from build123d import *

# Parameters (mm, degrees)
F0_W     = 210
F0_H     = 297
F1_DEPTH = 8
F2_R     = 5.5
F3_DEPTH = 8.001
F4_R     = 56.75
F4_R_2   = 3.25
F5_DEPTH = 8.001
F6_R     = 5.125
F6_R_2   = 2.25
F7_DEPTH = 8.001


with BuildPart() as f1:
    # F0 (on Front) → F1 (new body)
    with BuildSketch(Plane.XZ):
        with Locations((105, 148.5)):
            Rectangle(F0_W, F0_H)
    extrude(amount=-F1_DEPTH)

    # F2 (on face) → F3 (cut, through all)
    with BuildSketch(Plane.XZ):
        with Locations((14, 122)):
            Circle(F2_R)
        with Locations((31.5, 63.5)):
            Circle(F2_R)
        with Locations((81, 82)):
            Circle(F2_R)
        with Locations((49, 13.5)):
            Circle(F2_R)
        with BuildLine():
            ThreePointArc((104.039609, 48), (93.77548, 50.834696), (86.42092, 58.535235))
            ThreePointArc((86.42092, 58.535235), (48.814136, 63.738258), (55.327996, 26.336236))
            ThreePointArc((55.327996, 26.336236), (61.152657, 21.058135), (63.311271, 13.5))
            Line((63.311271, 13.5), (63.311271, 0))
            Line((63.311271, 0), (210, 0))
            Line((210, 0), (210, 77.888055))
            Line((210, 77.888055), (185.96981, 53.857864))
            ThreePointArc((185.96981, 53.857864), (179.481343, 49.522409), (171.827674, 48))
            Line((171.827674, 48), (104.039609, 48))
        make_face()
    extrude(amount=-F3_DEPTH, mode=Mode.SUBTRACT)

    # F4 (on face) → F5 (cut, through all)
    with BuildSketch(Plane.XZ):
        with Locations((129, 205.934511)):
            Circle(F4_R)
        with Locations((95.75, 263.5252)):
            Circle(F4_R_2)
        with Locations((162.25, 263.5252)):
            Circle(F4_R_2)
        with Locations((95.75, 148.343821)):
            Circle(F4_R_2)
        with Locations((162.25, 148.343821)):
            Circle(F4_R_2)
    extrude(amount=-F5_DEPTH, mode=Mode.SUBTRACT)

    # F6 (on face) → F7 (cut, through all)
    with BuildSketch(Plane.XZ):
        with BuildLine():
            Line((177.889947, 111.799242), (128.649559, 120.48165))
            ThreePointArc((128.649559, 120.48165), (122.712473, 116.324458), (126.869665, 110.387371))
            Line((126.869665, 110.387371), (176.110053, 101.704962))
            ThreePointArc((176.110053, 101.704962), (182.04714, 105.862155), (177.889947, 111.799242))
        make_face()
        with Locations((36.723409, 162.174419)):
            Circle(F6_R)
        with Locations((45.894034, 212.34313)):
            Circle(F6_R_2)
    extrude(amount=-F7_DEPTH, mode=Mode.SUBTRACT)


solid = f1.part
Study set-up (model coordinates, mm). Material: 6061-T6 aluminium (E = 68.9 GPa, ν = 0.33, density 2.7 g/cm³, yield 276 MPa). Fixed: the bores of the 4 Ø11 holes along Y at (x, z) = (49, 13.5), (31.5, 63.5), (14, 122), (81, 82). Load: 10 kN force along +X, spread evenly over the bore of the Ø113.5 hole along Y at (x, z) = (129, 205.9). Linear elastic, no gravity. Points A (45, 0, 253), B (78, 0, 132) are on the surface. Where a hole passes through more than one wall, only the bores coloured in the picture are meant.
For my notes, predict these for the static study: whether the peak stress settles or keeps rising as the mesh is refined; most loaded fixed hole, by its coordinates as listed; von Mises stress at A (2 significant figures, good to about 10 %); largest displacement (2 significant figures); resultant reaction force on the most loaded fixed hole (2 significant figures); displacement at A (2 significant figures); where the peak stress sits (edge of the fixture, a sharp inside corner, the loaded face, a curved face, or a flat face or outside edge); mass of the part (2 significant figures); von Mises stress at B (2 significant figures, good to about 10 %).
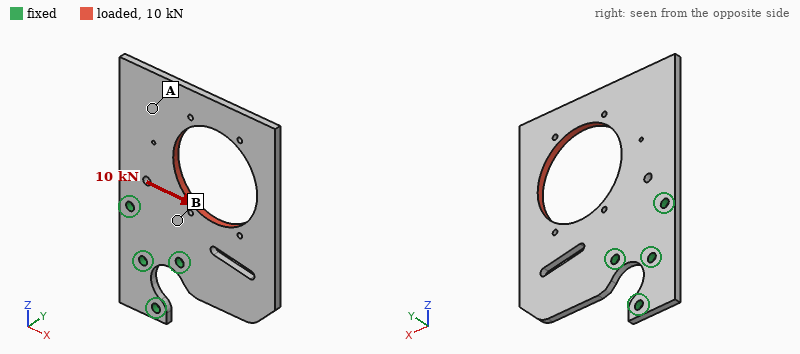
keeps rising
(14, 122)
9.8 MPa
0.32 mm
15 kN
0.21 mm
edge of the fixture
910 g
42 MPa
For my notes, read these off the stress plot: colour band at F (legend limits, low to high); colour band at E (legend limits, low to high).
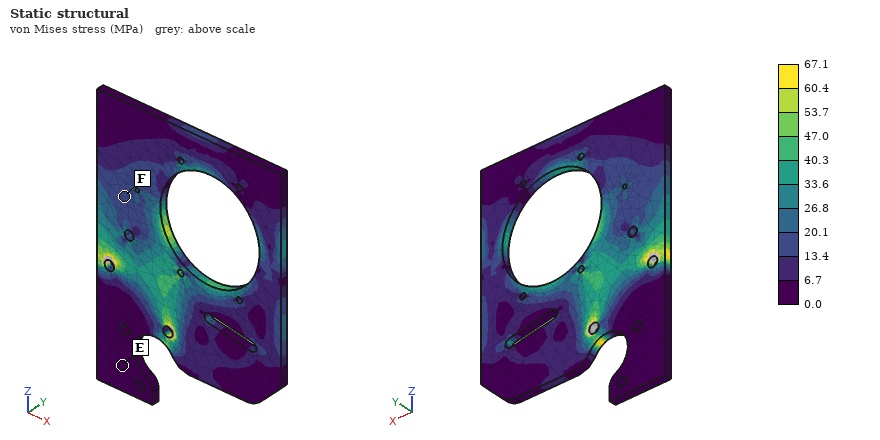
13.4 to 20.1 MPa
0.0 to 6.7 MPa
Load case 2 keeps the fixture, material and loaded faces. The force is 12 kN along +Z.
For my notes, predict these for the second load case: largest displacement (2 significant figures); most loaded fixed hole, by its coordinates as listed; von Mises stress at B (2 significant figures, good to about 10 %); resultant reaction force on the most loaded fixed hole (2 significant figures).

0.31 mm
(81, 82)
39 MPa
16 kN
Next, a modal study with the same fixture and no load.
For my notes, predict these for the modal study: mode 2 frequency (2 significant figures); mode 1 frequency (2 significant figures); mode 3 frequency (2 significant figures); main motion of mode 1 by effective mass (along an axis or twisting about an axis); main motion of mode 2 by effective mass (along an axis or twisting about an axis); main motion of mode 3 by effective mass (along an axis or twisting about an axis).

280 Hz
140 Hz
480 Hz
along Y
twisting about Z
along Y
